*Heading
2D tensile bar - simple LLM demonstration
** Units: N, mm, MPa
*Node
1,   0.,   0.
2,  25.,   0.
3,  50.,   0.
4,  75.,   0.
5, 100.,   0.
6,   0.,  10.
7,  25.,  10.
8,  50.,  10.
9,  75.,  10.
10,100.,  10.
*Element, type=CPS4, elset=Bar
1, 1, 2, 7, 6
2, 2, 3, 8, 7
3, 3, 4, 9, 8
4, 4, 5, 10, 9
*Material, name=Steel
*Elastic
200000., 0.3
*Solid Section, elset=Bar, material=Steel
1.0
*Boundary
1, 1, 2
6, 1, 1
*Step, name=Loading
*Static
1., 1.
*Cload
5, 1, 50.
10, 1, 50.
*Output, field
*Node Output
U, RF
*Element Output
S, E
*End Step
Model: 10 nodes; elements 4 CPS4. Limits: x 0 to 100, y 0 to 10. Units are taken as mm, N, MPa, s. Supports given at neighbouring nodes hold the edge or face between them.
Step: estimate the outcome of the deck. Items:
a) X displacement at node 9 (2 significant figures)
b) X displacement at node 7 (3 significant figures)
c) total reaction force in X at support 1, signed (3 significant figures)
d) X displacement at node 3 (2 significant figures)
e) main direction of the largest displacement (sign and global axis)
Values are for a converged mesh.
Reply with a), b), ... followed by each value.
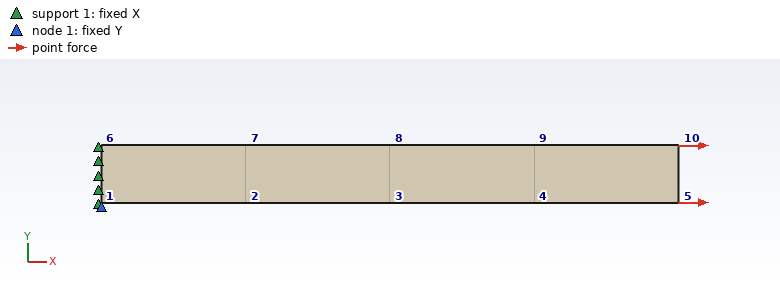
a) 0.0038 mm
b) 0.00125 mm
c) -100 N
d) 0.0025 mm
e) +X
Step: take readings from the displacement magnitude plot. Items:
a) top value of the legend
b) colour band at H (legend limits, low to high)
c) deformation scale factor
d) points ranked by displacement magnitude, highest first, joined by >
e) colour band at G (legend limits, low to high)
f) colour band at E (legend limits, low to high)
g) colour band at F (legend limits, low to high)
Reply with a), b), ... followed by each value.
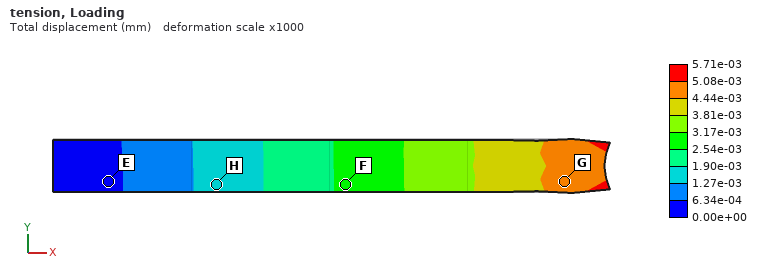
a) 5.71e-03 mm
b) 1.27e-03 to 1.90e-03 mm
c) 1000
d) G > F > H > E
e) 4.44e-03 to 5.08e-03 mm
f) 0.00e+00 to 6.34e-04 mm
g) 2.54e-03 to 3.17e-03 mm
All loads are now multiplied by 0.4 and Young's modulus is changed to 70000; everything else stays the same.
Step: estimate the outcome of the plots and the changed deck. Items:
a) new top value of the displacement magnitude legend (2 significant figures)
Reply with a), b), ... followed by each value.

a) 0.0065 mm
